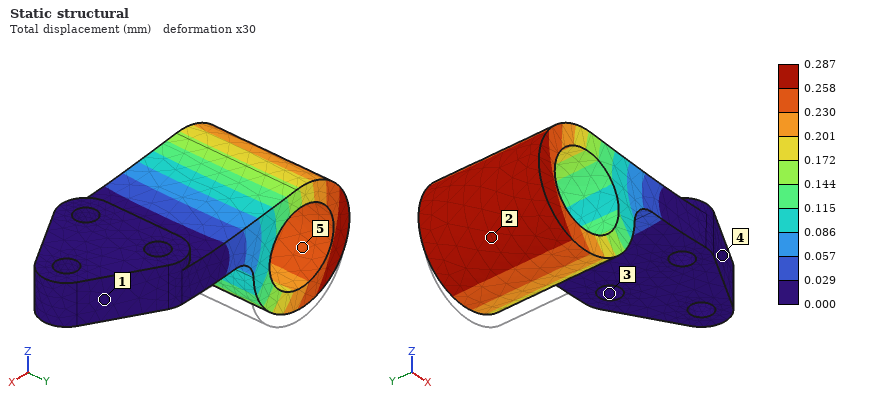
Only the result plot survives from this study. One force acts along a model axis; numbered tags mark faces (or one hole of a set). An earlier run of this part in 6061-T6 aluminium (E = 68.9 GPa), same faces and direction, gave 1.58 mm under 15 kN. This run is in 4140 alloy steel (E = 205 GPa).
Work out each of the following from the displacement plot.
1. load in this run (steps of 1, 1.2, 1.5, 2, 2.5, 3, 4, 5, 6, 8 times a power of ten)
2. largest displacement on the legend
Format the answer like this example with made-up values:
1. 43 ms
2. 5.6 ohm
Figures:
1. 8 kN
2. 0.287 mm
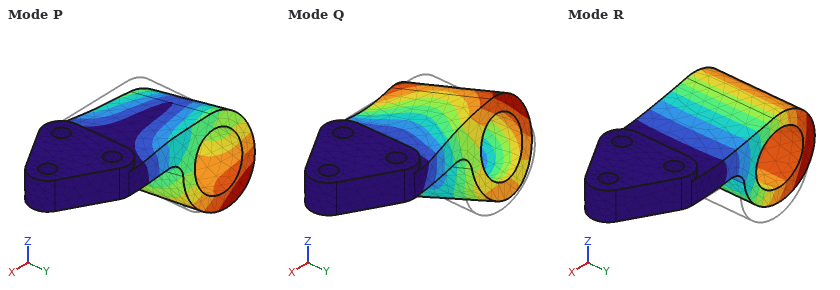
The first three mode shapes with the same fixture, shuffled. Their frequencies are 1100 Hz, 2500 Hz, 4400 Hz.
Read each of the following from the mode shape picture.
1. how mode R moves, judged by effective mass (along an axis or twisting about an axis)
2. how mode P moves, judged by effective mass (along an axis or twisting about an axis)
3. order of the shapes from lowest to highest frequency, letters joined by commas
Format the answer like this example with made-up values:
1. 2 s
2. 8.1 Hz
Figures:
1. along Z
2. along Y
3. R, P, Q
